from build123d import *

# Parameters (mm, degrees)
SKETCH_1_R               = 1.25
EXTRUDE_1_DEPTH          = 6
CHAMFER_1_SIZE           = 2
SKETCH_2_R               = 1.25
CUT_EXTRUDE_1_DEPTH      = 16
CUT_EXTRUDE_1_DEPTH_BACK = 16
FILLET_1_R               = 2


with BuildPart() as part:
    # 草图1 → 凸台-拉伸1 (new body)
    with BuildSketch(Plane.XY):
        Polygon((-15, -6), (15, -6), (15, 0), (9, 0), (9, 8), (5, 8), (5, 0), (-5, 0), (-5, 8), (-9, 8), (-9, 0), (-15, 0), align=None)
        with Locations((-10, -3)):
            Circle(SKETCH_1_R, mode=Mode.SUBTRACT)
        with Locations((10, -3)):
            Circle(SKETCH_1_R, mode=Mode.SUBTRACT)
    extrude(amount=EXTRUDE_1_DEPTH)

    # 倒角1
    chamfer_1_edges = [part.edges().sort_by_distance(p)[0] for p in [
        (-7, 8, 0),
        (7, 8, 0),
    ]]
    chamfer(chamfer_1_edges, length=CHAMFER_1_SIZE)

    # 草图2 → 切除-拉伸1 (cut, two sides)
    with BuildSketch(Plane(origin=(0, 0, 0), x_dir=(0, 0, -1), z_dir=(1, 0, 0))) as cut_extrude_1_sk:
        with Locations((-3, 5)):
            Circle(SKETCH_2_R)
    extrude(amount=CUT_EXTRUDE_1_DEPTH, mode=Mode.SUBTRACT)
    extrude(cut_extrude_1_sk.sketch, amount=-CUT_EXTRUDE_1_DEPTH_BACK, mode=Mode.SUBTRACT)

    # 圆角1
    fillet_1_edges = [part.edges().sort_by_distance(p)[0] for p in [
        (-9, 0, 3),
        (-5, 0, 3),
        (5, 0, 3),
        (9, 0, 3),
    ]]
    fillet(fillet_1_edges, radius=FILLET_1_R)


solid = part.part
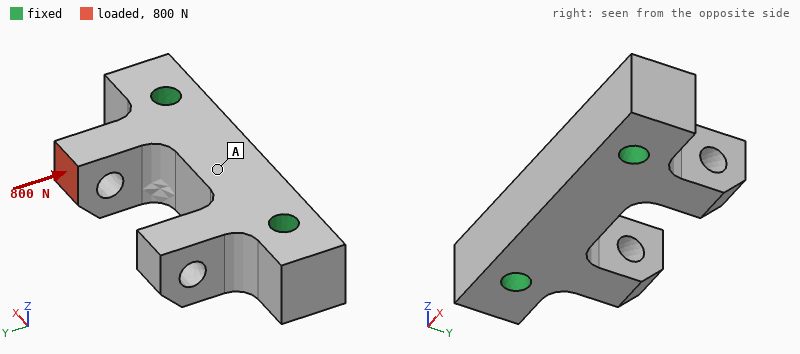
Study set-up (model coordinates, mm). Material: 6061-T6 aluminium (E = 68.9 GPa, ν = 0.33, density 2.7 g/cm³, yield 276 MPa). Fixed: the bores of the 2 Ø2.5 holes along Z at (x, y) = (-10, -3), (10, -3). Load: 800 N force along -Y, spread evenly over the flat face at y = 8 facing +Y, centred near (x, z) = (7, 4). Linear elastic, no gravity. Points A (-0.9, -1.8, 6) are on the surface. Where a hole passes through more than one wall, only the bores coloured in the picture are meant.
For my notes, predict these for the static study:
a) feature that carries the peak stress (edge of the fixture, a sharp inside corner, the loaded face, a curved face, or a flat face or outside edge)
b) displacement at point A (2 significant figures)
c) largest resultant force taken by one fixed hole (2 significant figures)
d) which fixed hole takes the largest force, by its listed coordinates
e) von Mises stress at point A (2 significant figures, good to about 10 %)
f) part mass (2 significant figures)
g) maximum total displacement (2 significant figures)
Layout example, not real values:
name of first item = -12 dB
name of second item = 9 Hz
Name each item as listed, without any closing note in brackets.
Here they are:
feature that carries the peak stress = a curved face
displacement at point A = 3.0 µm
largest resultant force taken by one fixed hole = 710 N
which fixed hole takes the largest force, by its listed coordinates = (10, -3)
von Mises stress at point A = 12 MPa
part mass = 3.7 g
maximum total displacement = 15 µm
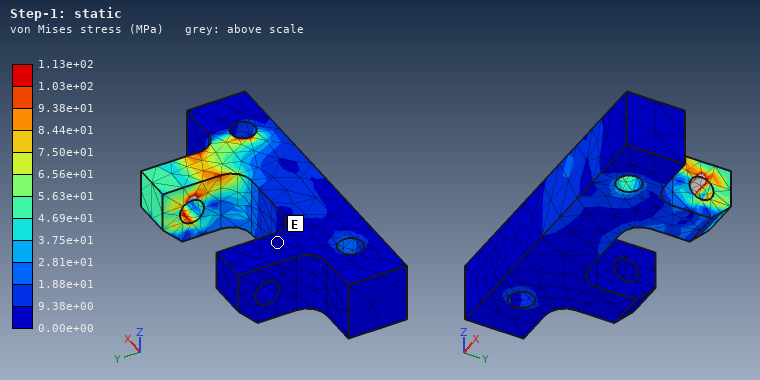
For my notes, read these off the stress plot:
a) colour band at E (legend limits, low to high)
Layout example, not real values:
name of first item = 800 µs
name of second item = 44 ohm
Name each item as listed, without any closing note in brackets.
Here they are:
colour band at E = 0.00e+00 to 9.38e+00 MPa
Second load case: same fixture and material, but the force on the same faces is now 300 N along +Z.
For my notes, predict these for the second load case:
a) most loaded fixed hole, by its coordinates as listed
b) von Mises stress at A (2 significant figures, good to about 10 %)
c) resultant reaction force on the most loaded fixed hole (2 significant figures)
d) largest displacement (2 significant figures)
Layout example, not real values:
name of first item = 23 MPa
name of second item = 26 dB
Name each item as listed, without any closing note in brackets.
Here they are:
most loaded fixed hole, by its coordinates as listed = (10, -3)
von Mises stress at A = 14 MPa
resultant reaction force on the most loaded fixed hole = 300 N
largest displacement = 36 µm
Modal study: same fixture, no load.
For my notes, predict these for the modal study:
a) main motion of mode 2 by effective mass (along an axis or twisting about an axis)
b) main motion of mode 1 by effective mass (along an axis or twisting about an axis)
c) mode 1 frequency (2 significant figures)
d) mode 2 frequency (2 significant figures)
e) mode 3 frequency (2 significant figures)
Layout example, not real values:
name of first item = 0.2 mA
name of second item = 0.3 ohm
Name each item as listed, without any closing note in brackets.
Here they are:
main motion of mode 2 by effective mass = along Z
main motion of mode 1 by effective mass = along Y
mode 1 frequency = 34 kHz
mode 2 frequency = 37 kHz
mode 3 frequency = 41 kHz
